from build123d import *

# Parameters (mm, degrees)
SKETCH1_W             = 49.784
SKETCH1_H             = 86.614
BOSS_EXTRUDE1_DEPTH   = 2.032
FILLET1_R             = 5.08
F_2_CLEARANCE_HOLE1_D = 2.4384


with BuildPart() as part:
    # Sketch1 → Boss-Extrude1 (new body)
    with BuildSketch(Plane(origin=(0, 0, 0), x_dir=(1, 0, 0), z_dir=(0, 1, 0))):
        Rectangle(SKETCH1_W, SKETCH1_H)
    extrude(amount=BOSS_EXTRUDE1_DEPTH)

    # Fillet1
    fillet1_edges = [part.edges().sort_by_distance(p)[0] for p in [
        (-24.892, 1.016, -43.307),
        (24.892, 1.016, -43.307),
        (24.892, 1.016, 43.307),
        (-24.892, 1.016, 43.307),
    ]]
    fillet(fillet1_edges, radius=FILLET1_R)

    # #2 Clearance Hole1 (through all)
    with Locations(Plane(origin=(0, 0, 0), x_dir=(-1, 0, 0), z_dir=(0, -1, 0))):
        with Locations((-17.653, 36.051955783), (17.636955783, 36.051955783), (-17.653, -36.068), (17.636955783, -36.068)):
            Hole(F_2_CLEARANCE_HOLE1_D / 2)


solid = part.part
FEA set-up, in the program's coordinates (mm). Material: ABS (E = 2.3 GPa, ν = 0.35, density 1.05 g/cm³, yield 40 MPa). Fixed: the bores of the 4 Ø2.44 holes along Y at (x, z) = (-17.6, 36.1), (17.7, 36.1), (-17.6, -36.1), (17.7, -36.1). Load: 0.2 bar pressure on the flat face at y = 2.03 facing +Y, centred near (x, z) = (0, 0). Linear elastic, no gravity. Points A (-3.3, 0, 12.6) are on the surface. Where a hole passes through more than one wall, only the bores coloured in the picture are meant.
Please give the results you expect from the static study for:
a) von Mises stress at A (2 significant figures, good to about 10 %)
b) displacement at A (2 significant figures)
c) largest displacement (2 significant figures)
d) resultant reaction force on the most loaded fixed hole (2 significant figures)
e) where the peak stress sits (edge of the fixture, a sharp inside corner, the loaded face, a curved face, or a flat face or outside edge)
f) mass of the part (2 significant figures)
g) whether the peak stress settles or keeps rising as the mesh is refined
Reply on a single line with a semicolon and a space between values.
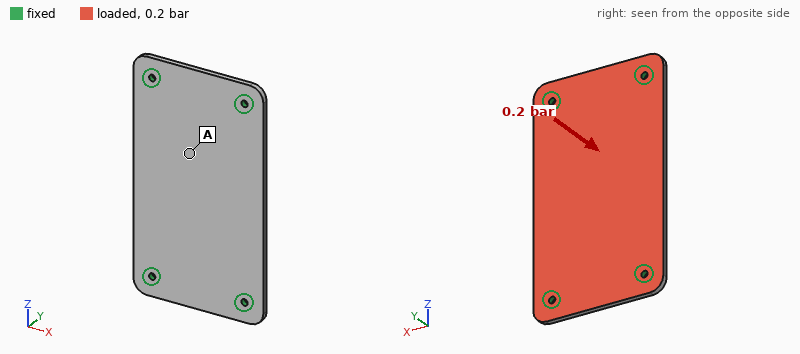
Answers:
4.1 MPa; 0.84 mm; 1.1 mm; 21 N; edge of the fixture; 9.1 g; keeps rising
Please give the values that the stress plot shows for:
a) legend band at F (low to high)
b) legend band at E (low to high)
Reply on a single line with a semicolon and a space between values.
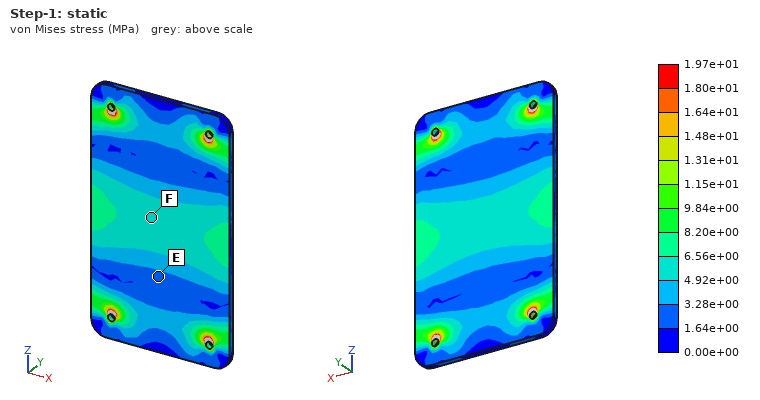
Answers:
4.92e+00 to 6.56e+00 MPa; 1.64e+00 to 3.28e+00 MPa
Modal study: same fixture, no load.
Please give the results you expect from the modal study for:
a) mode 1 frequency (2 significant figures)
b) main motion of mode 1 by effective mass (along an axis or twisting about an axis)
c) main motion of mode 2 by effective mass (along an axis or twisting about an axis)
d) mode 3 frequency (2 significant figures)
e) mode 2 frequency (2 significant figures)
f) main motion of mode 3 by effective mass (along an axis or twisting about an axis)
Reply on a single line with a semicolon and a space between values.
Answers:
540 Hz; along Y; twisting about Z; 1500 Hz; 810 Hz; twisting about X
